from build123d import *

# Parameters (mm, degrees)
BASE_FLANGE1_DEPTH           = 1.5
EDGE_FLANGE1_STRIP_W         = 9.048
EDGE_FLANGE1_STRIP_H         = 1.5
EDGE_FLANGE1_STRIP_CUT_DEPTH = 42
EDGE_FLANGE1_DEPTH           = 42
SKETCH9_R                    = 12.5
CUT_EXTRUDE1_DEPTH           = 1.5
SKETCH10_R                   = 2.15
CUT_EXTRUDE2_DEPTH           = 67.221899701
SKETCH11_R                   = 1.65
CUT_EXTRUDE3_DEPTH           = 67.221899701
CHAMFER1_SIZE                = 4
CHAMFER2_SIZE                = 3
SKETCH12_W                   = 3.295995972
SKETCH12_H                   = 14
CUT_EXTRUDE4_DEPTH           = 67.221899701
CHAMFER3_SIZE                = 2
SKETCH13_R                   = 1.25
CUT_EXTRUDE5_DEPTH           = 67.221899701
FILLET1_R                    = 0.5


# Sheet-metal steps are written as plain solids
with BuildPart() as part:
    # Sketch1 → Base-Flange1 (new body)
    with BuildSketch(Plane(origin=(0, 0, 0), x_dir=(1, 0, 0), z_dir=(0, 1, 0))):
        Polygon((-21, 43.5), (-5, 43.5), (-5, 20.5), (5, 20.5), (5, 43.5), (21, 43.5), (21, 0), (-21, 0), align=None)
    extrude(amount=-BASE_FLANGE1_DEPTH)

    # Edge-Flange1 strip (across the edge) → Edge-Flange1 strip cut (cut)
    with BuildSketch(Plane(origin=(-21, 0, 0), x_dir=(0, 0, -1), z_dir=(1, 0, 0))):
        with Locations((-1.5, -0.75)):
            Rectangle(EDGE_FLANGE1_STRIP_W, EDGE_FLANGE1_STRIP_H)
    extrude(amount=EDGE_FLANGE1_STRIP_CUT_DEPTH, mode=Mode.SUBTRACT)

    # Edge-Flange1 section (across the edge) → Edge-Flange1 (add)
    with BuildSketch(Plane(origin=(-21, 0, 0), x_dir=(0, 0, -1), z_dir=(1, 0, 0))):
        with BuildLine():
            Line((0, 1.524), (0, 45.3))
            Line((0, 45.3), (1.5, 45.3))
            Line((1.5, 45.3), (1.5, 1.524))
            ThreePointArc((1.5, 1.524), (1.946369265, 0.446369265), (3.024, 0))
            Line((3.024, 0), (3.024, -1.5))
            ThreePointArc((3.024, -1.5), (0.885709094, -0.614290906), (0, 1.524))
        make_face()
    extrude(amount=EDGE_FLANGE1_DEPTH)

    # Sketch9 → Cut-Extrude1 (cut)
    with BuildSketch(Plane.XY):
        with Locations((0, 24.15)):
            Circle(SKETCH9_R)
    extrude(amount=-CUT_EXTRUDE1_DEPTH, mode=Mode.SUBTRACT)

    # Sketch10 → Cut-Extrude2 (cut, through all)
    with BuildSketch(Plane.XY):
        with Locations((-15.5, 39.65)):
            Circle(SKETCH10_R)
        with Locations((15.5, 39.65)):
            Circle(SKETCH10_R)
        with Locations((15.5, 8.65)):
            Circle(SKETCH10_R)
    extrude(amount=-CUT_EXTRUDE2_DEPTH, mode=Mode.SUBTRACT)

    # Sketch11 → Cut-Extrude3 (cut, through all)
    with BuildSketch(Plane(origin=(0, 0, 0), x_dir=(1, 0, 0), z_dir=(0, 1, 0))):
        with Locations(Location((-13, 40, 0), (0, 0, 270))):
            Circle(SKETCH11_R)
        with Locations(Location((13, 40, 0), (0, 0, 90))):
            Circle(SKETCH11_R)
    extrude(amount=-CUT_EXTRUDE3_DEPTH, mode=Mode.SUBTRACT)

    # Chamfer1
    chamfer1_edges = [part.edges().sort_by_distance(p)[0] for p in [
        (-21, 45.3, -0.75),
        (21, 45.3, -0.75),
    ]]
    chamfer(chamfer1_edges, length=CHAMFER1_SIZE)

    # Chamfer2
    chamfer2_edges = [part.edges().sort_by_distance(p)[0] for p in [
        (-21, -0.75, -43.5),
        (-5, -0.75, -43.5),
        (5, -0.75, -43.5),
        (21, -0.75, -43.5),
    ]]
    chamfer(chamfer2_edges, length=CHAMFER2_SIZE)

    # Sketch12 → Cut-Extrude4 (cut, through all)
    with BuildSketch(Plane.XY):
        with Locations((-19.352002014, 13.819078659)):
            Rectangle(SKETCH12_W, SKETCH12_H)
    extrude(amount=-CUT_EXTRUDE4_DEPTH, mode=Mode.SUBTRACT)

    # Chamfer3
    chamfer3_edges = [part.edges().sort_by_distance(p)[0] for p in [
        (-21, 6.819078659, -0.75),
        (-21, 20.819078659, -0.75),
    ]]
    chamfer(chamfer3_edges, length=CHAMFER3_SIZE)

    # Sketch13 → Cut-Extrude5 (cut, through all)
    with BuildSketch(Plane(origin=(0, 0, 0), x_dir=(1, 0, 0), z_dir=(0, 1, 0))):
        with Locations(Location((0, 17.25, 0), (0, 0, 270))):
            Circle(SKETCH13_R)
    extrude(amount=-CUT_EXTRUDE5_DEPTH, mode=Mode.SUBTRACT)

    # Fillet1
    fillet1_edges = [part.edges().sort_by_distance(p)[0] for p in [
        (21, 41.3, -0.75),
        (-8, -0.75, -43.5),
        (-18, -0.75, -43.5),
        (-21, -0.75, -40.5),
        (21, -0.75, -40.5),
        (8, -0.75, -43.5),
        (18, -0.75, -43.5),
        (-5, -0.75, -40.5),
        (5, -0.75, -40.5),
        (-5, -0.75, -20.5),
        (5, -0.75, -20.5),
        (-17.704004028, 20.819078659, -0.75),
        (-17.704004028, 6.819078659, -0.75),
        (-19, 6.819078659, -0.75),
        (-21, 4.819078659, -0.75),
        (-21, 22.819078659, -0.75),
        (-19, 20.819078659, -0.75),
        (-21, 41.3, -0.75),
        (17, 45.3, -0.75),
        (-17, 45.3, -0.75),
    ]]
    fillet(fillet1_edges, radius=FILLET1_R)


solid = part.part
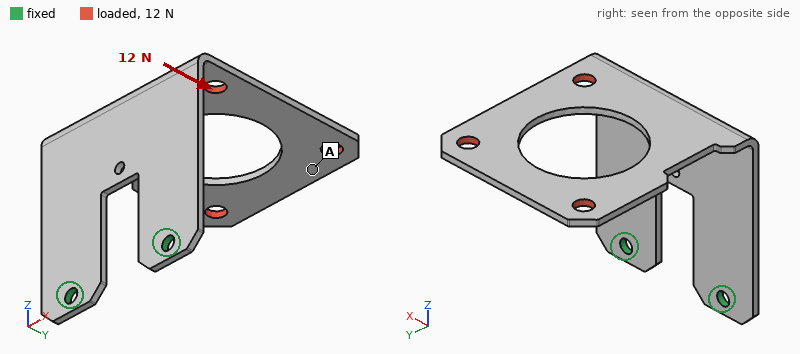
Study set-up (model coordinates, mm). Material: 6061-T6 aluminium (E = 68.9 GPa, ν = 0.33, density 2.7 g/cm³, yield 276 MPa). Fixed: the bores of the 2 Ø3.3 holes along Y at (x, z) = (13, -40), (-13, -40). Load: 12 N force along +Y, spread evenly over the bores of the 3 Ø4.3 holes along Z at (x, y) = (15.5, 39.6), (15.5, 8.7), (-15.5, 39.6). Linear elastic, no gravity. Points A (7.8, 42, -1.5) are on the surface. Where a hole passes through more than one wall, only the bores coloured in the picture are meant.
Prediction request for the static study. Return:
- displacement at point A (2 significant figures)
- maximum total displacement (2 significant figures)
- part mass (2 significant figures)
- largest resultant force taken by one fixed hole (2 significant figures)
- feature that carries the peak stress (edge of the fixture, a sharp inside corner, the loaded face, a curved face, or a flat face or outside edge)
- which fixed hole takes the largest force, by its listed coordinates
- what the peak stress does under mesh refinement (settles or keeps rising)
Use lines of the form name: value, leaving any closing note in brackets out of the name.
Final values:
displacement at point A: 0.69 mm
maximum total displacement: 0.75 mm
part mass: 11 g
largest resultant force taken by one fixed hole: 7.3 N
feature that carries the peak stress: edge of the fixture
which fixed hole takes the largest force, by its listed coordinates: (13, -40)
what the peak stress does under mesh refinement: keeps rising
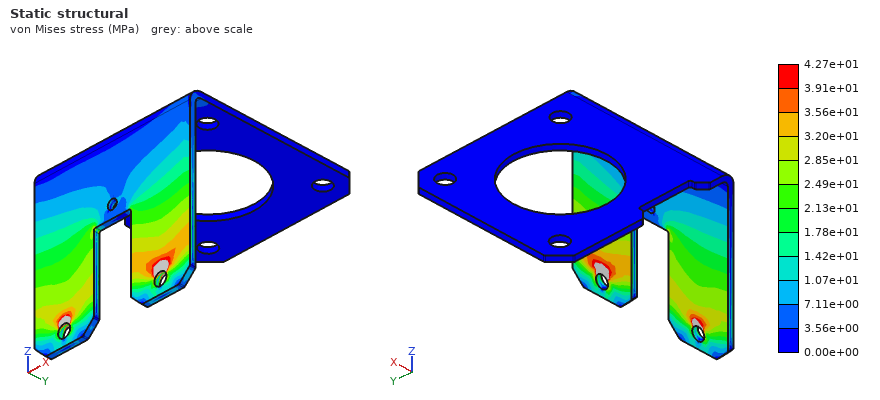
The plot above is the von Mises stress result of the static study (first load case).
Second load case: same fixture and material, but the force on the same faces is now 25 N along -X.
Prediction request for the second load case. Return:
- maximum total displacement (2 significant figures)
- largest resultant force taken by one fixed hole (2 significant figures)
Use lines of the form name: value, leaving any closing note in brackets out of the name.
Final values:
maximum total displacement: 0.87 mm
largest resultant force taken by one fixed hole: 35 N
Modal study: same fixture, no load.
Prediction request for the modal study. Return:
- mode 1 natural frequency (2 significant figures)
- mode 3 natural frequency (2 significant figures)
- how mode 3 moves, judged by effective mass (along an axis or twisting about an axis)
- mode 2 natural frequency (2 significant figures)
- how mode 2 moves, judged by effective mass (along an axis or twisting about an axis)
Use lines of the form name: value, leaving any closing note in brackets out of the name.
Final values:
mode 1 natural frequency: 240 Hz
mode 3 natural frequency: 630 Hz
how mode 3 moves, judged by effective mass: along Y
mode 2 natural frequency: 460 Hz
how mode 2 moves, judged by effective mass: along X
